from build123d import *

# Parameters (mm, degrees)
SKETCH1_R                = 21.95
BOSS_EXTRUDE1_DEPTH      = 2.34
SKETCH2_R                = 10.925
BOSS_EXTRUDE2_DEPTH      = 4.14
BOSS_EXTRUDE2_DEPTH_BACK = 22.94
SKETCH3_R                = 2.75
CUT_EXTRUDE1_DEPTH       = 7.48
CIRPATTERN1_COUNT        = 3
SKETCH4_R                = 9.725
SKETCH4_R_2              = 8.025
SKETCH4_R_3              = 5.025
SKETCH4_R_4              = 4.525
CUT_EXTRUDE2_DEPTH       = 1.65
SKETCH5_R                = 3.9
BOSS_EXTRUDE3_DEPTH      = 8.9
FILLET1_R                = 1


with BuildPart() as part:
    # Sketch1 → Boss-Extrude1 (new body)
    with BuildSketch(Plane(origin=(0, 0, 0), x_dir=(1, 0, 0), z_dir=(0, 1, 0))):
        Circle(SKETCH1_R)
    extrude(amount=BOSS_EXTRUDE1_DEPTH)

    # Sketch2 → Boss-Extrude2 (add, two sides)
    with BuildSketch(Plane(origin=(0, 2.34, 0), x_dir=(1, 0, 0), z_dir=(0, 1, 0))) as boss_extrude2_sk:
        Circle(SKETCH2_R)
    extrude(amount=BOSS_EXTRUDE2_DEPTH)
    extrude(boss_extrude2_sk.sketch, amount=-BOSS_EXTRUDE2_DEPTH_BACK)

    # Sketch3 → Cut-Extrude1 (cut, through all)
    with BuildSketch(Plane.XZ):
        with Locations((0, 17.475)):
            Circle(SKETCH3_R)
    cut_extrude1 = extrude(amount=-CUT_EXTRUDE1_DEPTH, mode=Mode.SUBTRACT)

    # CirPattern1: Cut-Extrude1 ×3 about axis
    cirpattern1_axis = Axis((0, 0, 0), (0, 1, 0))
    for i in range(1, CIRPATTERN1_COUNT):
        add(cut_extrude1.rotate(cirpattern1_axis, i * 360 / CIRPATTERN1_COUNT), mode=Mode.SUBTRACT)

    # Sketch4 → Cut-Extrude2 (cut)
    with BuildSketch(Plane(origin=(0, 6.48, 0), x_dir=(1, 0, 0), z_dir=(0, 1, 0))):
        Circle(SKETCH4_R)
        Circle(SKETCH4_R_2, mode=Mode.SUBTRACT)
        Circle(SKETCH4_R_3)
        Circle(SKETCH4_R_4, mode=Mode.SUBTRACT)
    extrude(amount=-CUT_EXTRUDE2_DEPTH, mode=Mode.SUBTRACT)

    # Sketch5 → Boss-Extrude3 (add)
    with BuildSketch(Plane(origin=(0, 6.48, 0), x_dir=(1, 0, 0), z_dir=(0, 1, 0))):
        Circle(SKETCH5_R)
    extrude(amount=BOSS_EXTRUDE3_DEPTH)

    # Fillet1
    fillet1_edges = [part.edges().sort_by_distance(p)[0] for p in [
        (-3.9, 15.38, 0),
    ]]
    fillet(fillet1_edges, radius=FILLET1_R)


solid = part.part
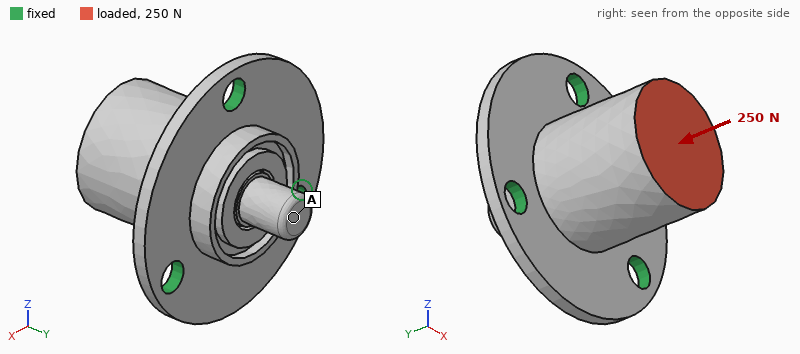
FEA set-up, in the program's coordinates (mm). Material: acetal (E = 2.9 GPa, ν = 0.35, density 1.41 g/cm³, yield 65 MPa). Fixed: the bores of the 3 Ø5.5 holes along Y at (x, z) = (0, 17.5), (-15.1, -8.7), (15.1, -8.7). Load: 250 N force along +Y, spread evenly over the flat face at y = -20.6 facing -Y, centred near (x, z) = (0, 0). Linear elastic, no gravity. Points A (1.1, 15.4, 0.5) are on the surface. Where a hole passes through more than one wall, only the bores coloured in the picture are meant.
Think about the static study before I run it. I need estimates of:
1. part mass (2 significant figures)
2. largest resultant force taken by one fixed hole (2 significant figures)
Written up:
18 g
84 N
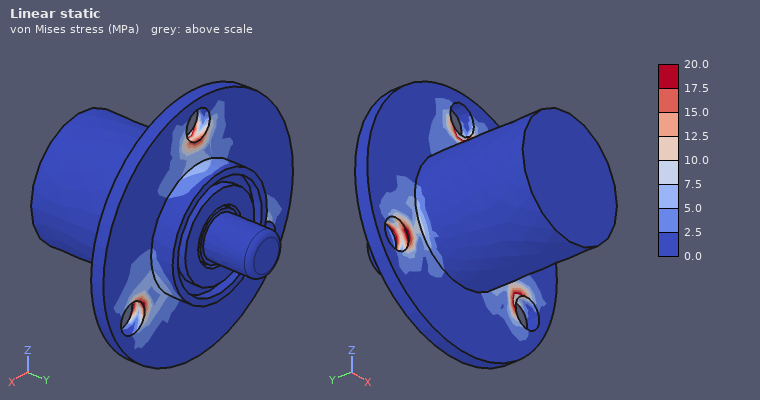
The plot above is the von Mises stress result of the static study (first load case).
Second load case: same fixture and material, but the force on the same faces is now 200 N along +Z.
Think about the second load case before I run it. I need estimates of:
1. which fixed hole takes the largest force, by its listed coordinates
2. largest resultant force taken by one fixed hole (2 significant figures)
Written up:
(0, 17.5)
220 N
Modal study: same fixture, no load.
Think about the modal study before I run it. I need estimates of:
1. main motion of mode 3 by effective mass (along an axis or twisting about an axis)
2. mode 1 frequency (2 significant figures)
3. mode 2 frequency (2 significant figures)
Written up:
along Y
2200 Hz
2200 Hz
